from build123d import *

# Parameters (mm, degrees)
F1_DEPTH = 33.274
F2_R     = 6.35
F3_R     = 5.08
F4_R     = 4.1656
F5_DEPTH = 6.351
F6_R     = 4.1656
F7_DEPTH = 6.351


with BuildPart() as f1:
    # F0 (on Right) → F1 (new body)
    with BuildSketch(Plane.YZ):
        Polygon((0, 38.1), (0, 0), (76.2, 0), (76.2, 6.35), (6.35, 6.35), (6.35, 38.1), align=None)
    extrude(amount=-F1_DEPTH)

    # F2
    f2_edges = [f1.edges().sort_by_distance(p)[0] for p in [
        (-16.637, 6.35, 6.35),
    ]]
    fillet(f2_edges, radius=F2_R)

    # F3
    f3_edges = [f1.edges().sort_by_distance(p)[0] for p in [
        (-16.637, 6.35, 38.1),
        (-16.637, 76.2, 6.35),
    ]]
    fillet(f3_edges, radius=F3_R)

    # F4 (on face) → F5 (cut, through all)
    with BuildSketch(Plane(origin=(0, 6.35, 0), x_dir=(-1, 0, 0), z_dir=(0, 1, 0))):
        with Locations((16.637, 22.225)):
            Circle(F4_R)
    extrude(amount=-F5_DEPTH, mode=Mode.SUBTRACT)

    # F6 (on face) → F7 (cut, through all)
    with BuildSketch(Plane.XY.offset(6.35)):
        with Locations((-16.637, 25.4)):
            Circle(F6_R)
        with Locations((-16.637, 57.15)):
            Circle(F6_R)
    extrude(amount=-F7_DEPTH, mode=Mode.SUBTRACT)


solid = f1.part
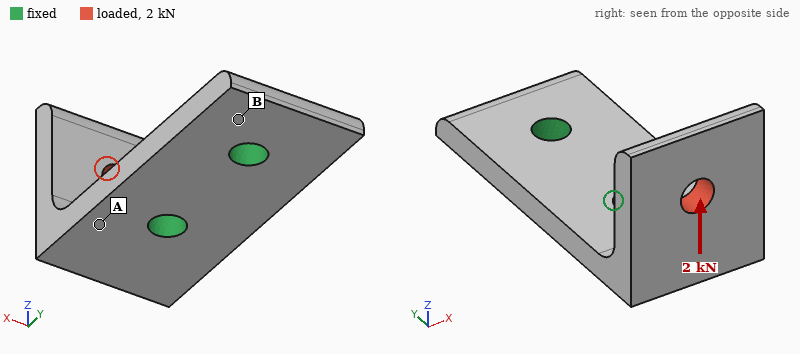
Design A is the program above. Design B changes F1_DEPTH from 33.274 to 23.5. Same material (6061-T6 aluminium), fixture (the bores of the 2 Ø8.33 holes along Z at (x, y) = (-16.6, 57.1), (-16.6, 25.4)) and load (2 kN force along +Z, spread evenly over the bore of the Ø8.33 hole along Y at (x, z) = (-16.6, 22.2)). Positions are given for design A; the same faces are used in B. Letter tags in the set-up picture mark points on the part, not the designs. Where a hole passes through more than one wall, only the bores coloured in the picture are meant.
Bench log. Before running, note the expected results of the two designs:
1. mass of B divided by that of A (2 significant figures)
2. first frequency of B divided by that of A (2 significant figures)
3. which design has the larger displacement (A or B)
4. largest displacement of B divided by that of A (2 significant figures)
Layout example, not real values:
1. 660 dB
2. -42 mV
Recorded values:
1. 0.69
2. 1.0
3. B
4. 1.4
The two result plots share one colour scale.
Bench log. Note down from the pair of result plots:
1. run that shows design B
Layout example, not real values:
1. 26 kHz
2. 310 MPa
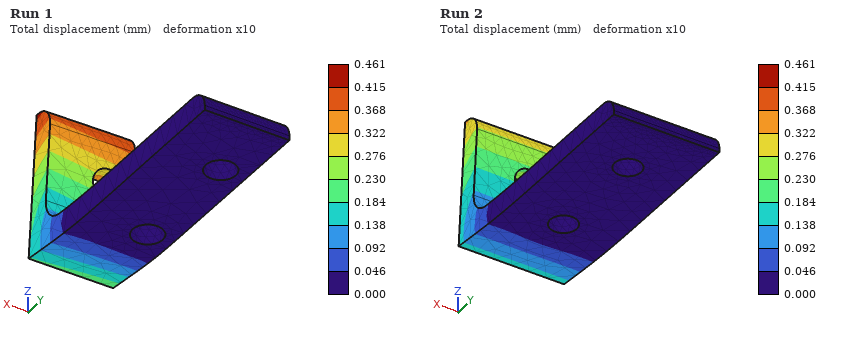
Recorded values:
1. Run 1
